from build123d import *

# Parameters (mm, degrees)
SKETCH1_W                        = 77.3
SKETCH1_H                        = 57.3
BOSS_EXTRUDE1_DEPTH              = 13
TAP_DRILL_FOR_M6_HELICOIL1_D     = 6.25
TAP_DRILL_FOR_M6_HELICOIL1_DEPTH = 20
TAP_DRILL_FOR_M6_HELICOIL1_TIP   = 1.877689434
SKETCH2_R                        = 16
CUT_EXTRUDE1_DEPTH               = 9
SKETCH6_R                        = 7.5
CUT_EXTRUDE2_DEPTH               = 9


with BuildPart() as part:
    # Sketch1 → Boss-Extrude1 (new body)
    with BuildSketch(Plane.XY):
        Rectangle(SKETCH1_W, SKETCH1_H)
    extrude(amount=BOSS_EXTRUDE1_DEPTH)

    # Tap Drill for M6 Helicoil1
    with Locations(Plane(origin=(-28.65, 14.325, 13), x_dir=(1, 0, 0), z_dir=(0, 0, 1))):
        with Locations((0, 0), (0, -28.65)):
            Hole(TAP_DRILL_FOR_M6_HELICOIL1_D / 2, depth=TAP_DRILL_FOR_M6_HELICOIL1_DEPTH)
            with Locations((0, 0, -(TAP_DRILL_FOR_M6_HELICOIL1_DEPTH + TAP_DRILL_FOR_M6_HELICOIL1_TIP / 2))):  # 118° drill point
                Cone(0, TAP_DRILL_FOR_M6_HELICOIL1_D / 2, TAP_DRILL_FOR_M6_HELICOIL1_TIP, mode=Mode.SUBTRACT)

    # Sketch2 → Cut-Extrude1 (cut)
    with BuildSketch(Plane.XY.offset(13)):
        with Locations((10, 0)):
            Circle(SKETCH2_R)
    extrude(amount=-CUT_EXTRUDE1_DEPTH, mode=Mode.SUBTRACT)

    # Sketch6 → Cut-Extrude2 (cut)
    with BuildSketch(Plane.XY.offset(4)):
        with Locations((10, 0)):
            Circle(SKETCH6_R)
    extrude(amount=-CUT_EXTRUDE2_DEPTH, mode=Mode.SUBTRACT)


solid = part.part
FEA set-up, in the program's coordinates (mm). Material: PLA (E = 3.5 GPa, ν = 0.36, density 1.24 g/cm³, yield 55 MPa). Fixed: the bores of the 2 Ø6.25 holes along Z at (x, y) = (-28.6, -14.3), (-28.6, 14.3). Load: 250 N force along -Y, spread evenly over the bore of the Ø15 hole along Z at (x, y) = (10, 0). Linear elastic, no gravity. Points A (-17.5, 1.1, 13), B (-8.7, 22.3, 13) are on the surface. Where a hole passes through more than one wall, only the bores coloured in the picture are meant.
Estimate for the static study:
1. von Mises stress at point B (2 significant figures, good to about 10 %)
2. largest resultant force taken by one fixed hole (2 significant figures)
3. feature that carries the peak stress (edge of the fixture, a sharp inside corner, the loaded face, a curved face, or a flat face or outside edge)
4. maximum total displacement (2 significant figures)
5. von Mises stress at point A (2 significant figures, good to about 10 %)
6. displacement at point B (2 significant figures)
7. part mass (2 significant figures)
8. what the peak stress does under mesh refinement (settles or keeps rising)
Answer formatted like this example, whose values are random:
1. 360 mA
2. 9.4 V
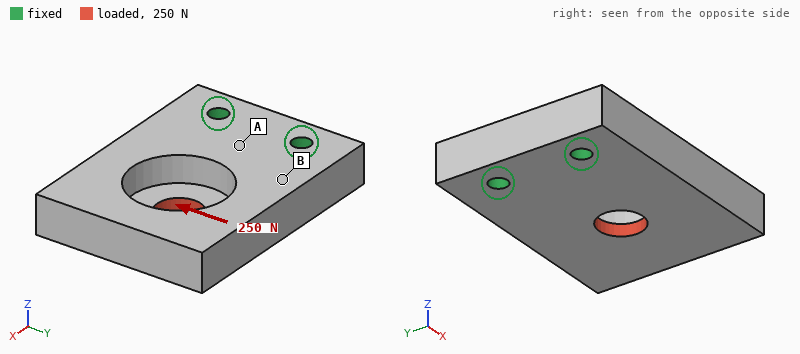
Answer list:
1. 0.57 MPa
2. 310 N
3. edge of the fixture
4. 58 µm
5. 1.2 MPa
6. 15 µm
7. 61 g
8. keeps rising
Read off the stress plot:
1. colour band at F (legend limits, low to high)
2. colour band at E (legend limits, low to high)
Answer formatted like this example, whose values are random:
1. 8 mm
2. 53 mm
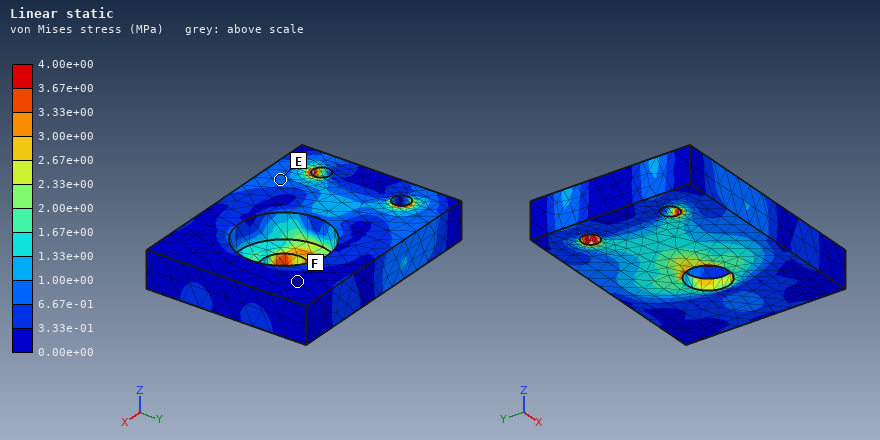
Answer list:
1. 0.00e+00 to 3.33e-01 MPa
2. 6.67e-01 to 1.00e+00 MPa
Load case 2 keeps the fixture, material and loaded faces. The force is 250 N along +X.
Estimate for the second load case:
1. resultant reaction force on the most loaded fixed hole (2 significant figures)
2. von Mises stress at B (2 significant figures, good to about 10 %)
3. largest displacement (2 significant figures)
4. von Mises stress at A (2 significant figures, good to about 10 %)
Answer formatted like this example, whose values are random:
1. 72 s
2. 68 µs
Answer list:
1. 130 N
2. 0.31 MPa
3. 59 µm
4. 0.36 MPa
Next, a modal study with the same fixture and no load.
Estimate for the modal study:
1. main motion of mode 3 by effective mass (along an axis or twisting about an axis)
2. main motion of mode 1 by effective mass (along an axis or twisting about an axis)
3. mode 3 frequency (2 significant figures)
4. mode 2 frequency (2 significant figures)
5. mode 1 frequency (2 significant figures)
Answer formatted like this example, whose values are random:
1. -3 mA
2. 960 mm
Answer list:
1. along Y
2. along Z
3. 1900 Hz
4. 1600 Hz
5. 730 Hz
